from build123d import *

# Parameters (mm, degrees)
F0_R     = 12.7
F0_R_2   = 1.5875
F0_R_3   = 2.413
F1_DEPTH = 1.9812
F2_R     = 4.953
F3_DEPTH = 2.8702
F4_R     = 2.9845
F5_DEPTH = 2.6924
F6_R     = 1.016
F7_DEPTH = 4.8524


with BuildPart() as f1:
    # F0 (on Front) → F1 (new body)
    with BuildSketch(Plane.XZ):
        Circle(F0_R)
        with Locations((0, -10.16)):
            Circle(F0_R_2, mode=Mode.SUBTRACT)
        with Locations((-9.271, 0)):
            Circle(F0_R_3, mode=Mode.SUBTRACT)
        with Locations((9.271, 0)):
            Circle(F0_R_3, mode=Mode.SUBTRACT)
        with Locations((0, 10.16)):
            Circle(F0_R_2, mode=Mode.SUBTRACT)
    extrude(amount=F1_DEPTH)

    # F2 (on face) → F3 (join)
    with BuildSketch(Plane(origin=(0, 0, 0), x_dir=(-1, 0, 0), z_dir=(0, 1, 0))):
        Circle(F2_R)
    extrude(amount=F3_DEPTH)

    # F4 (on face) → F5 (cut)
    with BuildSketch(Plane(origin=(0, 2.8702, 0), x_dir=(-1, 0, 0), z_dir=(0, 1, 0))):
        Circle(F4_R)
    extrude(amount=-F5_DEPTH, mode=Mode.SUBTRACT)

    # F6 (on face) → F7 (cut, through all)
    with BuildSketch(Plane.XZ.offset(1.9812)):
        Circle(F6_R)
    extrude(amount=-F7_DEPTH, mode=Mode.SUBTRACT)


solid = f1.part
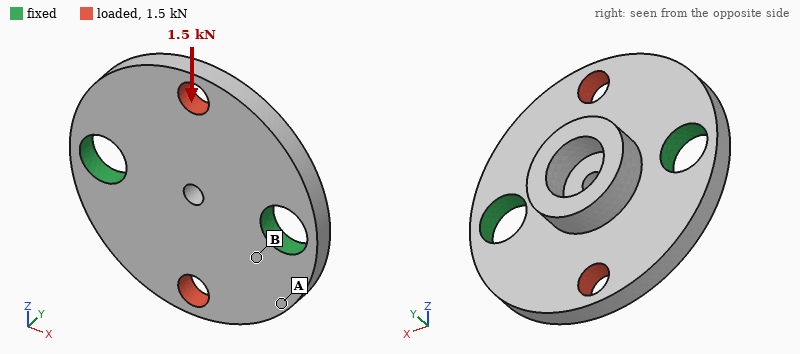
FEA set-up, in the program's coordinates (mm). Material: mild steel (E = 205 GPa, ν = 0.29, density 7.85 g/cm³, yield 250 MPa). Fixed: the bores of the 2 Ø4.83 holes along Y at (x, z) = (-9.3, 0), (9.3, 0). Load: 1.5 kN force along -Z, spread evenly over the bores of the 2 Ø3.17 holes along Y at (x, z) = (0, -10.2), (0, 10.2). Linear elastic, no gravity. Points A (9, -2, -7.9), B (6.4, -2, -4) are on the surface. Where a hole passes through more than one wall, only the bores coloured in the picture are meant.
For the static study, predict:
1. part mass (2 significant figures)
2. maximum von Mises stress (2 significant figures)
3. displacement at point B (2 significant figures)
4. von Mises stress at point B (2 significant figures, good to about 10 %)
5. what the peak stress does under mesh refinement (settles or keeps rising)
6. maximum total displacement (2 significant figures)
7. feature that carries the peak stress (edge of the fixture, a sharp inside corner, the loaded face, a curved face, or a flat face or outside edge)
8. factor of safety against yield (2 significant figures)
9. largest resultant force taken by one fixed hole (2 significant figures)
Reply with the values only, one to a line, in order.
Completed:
8.2 g
140 MPa
0.61 µm
41 MPa
settles
3.9 µm
a curved face
1.8
750 N
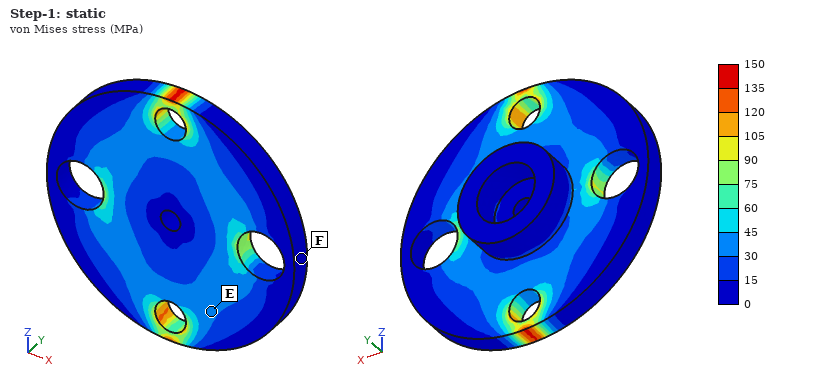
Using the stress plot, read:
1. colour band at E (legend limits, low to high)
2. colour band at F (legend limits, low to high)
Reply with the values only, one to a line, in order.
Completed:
30 to 45 MPa
0 to 15 MPa
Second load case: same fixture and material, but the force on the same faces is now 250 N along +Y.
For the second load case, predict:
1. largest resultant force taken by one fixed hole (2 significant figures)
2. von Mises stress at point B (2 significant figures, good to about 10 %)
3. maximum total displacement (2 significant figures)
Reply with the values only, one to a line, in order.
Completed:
140 N
37 MPa
15 µm
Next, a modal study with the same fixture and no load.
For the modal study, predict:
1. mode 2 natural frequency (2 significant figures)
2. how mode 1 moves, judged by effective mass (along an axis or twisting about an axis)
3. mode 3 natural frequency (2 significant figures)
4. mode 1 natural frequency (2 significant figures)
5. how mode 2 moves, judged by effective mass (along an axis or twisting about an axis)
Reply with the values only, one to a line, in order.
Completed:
19 kHz
twisting about X
34 kHz
15 kHz
along Y
